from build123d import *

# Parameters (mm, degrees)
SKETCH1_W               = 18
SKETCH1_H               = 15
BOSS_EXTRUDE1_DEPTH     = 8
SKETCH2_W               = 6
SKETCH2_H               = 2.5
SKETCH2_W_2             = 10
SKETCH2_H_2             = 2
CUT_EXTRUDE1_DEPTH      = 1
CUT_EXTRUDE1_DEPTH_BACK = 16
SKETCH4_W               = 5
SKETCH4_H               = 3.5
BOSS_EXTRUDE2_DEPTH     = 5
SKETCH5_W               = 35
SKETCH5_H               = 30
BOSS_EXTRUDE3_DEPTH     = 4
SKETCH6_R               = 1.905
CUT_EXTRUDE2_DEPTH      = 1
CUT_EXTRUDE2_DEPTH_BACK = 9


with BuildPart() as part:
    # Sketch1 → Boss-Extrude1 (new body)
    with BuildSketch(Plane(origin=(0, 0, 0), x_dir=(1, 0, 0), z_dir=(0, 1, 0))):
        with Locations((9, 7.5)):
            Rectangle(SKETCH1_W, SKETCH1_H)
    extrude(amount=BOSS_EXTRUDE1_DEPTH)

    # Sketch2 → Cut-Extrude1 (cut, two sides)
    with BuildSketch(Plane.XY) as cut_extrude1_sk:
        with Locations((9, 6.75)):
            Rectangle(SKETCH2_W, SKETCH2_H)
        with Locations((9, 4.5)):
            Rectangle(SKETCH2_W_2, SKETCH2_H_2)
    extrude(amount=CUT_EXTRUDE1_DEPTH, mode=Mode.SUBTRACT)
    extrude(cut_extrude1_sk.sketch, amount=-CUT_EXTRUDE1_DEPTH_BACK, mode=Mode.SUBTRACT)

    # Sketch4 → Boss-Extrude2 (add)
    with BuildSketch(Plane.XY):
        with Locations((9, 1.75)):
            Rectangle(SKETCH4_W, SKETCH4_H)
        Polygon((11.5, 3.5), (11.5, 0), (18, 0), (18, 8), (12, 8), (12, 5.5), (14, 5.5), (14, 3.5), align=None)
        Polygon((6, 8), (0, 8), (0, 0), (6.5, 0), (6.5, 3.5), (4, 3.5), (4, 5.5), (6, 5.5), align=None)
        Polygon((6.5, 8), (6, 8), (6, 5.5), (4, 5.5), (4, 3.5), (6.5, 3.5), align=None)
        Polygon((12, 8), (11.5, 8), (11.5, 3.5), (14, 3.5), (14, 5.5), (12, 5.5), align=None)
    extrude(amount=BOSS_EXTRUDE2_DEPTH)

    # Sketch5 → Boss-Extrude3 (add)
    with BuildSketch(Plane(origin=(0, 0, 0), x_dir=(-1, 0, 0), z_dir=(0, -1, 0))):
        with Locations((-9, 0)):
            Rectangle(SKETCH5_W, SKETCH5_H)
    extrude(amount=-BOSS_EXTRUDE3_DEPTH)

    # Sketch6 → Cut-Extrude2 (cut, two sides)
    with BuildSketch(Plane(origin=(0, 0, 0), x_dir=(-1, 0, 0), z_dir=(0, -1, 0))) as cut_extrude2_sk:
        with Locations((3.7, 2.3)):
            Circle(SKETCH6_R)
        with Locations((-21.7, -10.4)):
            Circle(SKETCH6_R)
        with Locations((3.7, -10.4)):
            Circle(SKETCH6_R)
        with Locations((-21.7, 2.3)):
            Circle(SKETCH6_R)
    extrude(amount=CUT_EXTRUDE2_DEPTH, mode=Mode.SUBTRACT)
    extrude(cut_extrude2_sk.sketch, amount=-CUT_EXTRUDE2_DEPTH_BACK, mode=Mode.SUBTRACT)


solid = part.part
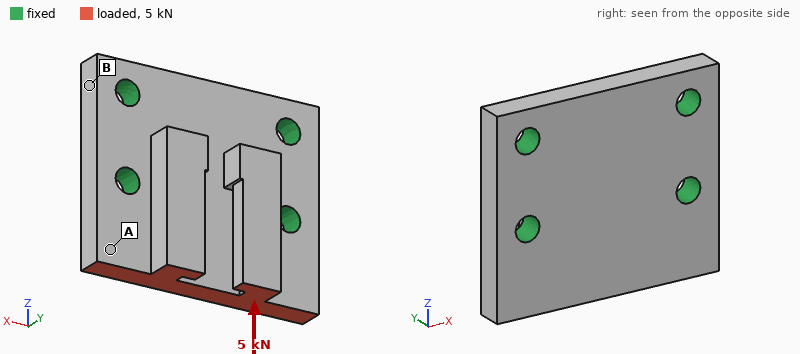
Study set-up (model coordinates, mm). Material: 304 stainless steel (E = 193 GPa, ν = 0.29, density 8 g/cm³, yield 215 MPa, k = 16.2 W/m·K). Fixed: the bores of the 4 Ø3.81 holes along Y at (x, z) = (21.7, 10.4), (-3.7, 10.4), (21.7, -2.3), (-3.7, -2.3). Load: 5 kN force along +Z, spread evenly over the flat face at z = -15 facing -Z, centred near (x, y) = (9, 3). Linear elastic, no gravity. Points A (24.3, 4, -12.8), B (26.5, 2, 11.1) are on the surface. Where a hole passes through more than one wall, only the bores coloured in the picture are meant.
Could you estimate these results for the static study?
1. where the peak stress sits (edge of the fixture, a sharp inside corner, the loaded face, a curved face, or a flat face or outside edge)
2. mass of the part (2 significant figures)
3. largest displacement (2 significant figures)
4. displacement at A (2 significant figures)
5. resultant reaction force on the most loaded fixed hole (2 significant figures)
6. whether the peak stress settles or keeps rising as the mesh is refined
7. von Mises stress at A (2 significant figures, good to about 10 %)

edge of the fixture
39 g
5.5 µm
2.6 µm
2.0 kN
keeps rising
29 MPa
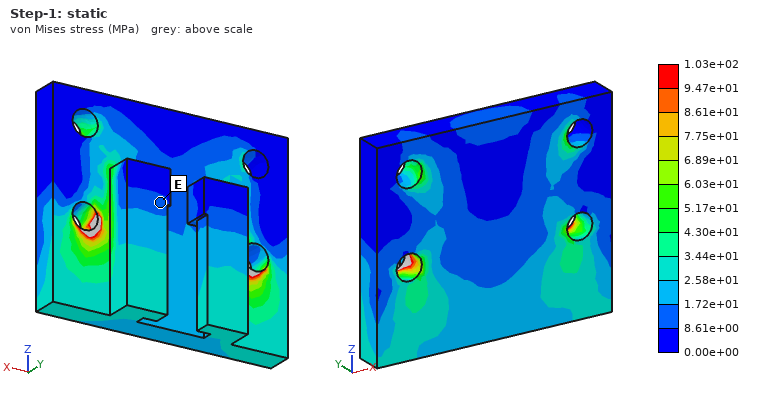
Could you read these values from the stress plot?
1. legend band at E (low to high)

8.61e+00 to 1.72e+01 MPa
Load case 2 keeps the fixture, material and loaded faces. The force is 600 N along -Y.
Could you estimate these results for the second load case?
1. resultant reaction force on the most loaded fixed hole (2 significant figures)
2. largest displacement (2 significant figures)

460 N
9.8 µm
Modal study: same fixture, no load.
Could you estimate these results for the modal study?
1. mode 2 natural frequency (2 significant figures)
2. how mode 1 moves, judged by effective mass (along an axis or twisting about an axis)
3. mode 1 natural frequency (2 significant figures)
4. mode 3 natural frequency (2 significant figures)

26 kHz
along Y
16 kHz
27 kHz
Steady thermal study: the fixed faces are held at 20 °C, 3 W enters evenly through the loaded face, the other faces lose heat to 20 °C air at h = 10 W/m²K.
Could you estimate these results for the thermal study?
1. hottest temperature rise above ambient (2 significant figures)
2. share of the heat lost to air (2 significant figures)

16 K
4.7 %
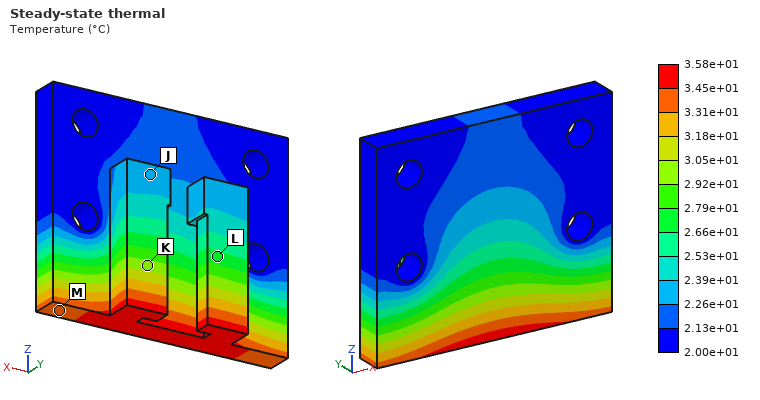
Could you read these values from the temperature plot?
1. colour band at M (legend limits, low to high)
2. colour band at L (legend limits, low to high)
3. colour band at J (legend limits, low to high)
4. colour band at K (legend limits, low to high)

3.31e+01 to 3.45e+01 °C
2.66e+01 to 2.79e+01 °C
2.26e+01 to 2.39e+01 °C
2.92e+01 to 3.05e+01 °C
